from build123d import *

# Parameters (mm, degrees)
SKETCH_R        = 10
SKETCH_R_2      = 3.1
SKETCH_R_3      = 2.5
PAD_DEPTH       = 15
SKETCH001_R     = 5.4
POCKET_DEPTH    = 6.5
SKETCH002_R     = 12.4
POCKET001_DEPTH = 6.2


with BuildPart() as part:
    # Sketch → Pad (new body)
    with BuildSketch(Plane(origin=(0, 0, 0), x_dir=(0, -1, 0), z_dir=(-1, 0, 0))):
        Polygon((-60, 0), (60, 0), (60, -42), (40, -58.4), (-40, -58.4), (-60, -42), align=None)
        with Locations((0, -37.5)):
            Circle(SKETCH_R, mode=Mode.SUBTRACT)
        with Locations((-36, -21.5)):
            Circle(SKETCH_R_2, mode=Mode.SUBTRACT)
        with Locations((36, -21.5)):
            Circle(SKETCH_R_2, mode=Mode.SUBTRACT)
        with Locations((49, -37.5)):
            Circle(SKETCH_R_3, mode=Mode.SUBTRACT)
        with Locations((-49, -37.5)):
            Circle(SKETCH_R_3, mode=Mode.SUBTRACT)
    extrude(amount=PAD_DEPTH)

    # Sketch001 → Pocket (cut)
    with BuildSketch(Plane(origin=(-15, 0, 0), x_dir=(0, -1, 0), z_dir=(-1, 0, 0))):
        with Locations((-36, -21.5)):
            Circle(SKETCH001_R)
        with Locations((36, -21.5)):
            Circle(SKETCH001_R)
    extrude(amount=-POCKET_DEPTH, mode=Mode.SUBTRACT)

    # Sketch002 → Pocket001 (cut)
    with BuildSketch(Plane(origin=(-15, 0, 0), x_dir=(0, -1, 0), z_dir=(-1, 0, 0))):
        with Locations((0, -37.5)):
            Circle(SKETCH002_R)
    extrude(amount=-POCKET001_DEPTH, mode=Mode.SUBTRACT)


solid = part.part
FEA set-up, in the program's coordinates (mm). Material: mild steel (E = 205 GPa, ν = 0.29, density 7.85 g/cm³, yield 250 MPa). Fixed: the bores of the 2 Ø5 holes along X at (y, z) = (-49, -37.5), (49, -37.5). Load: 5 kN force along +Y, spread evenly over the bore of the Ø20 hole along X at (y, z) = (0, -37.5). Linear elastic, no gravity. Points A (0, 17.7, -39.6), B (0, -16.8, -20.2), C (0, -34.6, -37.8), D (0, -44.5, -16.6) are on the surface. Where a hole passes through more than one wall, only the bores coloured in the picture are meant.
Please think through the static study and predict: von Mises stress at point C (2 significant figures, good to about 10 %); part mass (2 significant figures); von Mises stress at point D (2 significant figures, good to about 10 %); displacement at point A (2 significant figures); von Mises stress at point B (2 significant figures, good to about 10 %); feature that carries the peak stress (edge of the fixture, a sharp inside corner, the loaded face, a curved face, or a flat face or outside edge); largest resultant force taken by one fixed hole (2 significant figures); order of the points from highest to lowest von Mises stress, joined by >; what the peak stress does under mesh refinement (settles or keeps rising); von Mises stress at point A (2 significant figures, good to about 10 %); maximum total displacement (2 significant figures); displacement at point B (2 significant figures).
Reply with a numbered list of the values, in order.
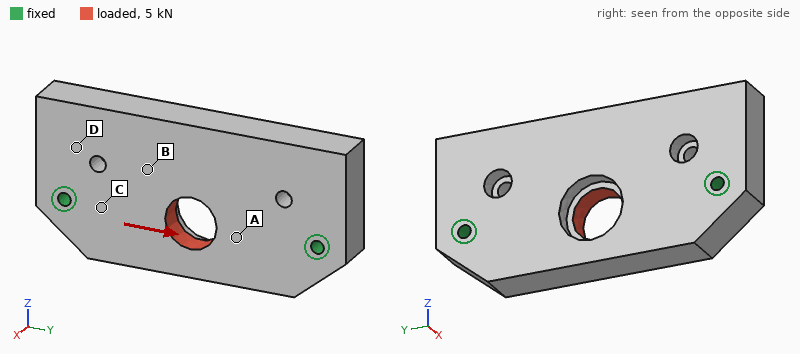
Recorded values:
1. 8.1 MPa
2. 720 g
3. 1.6 MPa
4. 1.2 µm
5. 3.3 MPa
6. edge of the fixture
7. 2.5 kN
8. A > C > B > D
9. keeps rising
10. 9.9 MPa
11. 1.7 µm
12. 1.1 µm
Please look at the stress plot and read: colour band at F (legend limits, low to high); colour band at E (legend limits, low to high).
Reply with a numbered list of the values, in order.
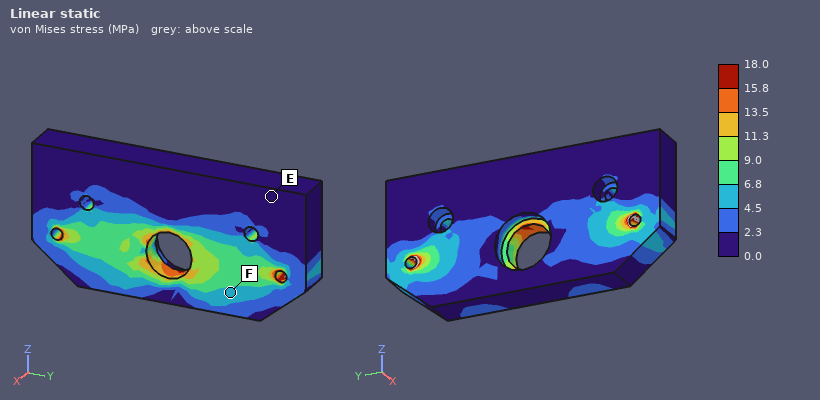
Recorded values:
1. 4.5 to 6.8 MPa
2. 0.0 to 2.3 MPa
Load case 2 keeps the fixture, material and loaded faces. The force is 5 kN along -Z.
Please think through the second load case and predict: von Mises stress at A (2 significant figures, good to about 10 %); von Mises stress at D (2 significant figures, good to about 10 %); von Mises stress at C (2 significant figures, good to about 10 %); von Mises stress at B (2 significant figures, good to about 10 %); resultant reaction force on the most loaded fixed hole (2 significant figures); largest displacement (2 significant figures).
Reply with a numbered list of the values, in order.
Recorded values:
1. 9.0 MPa
2. 5.9 MPa
3. 11 MPa
4. 9.3 MPa
5. 2.6 kN
6. 6.0 µm
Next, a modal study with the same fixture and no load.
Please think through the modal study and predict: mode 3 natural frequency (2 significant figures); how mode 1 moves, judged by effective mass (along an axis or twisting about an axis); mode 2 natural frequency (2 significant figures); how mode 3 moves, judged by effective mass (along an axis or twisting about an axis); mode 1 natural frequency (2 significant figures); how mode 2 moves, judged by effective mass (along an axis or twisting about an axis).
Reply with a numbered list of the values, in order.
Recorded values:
1. 7800 Hz
2. along X
3. 6400 Hz
4. twisting about Z
5. 4100 Hz
6. along X
